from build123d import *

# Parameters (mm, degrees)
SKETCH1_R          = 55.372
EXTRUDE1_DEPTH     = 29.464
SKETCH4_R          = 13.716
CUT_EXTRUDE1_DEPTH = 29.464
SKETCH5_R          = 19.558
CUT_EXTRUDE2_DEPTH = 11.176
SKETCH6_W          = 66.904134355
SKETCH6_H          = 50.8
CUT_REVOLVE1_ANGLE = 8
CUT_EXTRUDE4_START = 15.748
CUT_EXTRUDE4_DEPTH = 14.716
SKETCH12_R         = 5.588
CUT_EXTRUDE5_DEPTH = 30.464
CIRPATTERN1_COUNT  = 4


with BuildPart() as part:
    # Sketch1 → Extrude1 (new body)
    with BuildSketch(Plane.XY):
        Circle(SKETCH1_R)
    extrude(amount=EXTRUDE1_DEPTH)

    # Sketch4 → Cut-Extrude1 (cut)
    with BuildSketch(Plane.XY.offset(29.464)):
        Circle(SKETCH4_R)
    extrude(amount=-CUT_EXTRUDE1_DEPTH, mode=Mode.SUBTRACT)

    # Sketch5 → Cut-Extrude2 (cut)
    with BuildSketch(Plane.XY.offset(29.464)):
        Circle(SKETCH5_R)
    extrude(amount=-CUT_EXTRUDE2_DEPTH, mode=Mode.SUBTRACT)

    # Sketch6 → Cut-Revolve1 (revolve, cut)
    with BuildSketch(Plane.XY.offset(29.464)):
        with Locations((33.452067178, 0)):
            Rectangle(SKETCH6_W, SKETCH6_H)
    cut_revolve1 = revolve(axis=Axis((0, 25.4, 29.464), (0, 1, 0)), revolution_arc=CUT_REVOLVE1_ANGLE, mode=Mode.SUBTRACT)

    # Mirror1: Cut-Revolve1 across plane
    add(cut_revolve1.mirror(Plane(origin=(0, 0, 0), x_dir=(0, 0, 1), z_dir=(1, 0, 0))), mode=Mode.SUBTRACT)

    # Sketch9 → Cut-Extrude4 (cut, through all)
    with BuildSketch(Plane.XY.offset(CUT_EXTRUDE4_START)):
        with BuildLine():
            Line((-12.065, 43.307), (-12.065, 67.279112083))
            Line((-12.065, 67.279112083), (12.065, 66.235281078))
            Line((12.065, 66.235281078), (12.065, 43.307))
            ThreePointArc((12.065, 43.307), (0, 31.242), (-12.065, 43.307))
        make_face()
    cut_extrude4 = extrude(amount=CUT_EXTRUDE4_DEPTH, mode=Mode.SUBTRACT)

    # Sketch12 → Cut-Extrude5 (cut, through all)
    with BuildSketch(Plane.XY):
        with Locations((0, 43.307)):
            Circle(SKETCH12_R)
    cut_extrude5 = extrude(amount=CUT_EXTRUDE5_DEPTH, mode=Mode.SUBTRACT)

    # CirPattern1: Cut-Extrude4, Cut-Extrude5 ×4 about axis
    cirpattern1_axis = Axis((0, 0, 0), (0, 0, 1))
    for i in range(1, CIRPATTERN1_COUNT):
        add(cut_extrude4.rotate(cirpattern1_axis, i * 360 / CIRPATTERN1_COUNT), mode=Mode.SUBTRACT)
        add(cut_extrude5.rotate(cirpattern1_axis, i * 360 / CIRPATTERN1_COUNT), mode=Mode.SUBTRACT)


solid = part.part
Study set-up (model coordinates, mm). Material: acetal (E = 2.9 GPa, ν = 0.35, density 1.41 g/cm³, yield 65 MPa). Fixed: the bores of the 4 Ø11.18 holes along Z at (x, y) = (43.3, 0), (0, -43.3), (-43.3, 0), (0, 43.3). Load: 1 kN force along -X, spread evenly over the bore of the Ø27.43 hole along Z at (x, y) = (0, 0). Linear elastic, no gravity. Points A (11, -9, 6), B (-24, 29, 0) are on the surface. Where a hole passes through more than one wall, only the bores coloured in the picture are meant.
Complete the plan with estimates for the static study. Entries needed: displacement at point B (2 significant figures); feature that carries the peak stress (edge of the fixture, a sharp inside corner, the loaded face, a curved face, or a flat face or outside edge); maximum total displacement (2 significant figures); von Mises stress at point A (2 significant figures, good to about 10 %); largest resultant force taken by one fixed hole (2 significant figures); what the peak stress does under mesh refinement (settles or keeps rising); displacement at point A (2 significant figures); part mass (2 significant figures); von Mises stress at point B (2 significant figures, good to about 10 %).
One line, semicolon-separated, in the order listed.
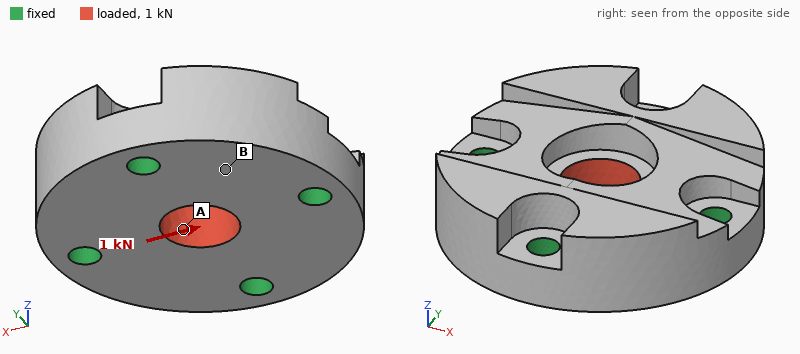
3.3 µm; edge of the fixture; 7.9 µm; 0.78 MPa; 320 N; keeps rising; 7.3 µm; 300 g; 0.19 MPa
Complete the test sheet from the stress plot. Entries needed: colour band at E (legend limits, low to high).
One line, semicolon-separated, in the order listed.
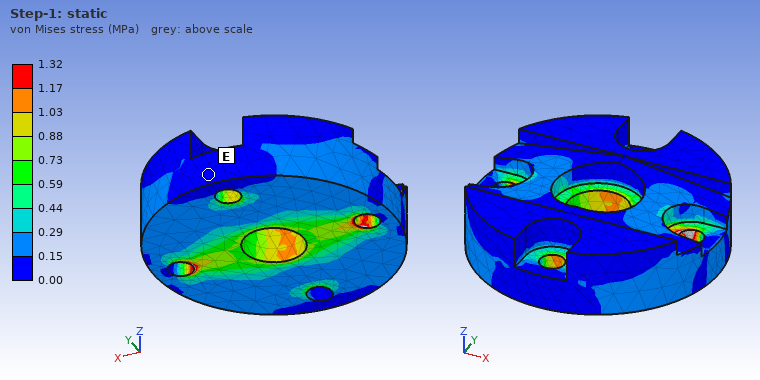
0.00 to 0.15 MPa
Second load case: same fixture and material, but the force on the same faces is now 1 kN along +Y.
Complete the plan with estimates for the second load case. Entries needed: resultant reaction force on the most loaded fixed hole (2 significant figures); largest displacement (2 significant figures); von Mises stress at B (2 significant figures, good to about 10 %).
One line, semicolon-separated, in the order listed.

320 N; 7.9 µm; 0.18 MPa
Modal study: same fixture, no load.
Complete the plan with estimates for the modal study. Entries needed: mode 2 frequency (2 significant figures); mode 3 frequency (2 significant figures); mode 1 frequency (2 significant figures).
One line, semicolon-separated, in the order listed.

3600 Hz; 3700 Hz; 3400 Hz
